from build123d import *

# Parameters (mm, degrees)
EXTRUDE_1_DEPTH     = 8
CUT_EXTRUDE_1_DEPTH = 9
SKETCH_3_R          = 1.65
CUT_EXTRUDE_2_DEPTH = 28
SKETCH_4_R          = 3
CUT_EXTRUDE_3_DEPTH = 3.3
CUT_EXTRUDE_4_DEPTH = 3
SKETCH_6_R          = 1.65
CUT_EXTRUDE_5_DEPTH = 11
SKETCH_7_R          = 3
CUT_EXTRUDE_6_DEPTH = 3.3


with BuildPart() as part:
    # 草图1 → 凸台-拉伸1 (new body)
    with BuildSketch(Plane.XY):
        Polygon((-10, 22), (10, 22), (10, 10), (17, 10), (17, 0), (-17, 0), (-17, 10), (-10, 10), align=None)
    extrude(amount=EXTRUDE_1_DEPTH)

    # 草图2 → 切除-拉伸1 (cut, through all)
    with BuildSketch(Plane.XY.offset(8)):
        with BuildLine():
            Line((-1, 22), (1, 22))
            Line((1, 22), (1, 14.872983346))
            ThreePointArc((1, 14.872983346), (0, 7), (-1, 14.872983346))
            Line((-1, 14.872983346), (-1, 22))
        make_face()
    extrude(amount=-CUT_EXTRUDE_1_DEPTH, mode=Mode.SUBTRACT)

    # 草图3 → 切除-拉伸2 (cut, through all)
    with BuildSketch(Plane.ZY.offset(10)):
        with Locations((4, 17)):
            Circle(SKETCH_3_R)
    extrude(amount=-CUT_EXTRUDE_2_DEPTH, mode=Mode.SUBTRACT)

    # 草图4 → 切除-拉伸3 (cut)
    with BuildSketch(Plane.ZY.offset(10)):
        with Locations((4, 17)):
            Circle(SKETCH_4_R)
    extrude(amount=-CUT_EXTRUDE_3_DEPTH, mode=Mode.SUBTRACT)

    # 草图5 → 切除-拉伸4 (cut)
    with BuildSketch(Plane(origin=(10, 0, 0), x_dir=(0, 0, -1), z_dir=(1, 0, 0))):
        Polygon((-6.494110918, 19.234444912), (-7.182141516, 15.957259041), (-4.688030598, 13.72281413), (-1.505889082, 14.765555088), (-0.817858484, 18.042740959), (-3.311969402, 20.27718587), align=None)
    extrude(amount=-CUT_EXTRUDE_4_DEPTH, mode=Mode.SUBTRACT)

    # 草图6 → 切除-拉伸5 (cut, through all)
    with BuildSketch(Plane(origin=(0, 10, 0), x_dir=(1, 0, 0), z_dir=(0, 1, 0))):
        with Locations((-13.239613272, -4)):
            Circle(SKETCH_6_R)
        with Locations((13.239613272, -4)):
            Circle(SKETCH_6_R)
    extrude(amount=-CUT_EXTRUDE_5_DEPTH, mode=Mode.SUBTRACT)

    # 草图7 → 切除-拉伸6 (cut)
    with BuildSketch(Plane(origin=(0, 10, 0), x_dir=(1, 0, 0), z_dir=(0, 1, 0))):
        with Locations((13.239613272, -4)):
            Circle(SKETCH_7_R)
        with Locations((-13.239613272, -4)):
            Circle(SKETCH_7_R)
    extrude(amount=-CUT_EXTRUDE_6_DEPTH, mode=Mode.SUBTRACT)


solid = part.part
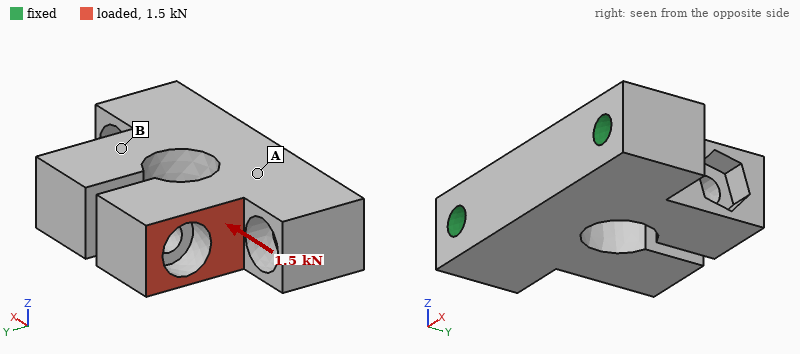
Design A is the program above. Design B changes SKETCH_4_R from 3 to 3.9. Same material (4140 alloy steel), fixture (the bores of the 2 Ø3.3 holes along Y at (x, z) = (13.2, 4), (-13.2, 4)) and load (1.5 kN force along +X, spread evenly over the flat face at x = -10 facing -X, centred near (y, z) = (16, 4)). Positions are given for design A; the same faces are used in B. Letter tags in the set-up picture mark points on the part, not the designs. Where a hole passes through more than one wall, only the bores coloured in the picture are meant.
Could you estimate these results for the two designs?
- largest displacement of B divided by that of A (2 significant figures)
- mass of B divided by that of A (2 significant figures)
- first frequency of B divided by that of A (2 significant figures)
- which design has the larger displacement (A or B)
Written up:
1.1
0.98
1.0
B
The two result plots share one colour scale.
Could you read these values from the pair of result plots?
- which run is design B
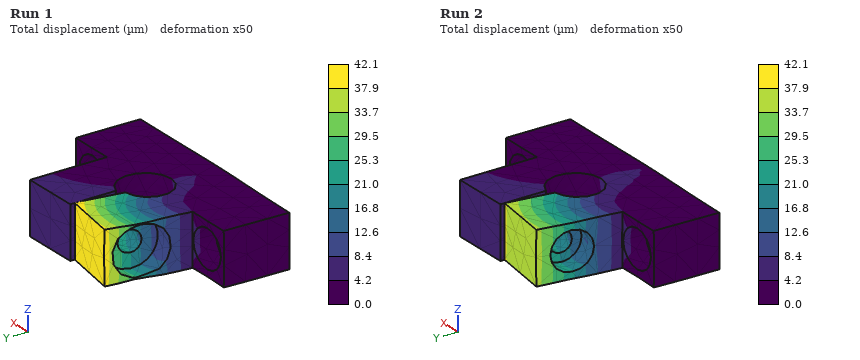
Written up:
Run 1
